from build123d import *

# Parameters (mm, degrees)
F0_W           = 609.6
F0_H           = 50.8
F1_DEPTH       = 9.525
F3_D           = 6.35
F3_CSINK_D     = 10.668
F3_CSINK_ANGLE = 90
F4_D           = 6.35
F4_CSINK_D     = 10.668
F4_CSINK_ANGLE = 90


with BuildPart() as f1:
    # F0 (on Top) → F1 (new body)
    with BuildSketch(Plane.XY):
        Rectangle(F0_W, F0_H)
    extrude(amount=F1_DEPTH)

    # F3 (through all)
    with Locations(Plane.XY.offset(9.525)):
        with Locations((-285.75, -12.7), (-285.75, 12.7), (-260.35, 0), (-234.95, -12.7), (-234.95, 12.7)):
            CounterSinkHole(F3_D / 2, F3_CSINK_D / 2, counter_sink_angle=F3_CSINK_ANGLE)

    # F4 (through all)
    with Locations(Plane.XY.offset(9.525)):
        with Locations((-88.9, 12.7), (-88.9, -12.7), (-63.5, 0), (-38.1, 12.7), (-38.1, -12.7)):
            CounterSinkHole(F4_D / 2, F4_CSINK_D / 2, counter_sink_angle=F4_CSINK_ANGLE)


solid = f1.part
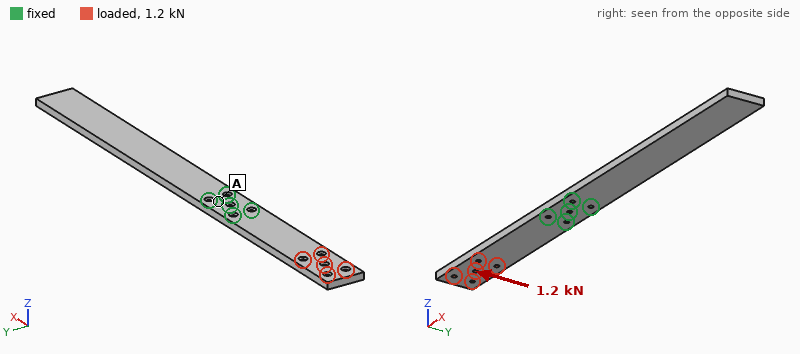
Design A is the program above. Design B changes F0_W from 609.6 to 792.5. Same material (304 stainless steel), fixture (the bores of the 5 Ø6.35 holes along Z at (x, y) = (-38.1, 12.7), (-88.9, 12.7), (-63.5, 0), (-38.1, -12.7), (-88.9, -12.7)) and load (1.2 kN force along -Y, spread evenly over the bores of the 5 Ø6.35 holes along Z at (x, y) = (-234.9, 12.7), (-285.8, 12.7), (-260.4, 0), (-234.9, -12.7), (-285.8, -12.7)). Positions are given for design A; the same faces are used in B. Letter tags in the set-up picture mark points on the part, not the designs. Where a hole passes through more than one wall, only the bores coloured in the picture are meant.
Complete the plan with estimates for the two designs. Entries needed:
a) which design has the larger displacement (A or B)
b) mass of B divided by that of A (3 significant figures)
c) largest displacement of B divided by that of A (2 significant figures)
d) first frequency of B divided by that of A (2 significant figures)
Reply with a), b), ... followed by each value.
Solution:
a) B
b) 1.30
c) 1.5
d) 0.62
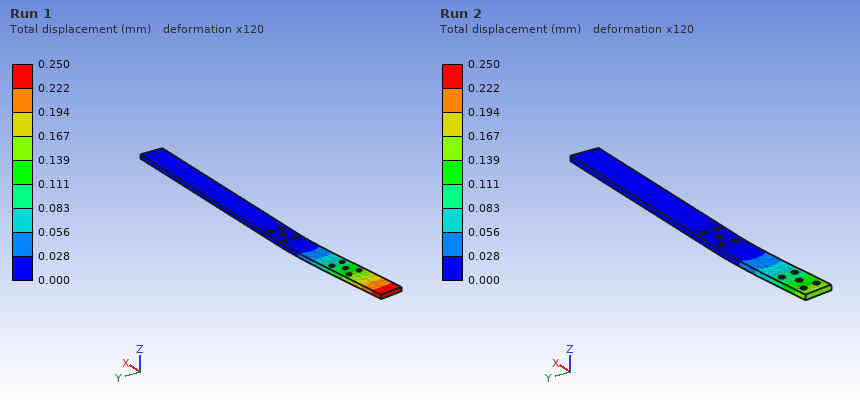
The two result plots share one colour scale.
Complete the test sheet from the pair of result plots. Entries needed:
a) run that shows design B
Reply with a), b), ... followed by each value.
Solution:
a) Run 1
